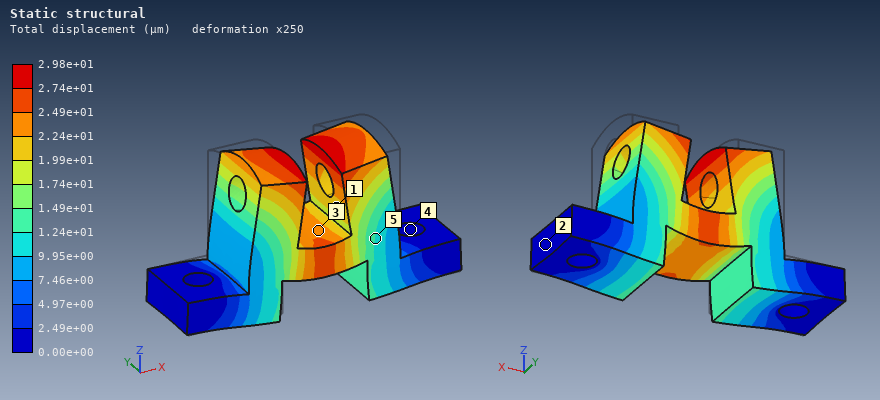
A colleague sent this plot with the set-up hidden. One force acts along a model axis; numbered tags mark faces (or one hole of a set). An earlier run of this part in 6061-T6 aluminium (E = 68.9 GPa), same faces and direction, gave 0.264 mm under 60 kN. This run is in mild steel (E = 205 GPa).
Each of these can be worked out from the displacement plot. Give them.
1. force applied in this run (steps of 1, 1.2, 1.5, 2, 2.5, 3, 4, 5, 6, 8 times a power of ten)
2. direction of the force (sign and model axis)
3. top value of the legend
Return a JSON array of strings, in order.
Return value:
["20 kN", "-Z", "2.98e+01 µm"]
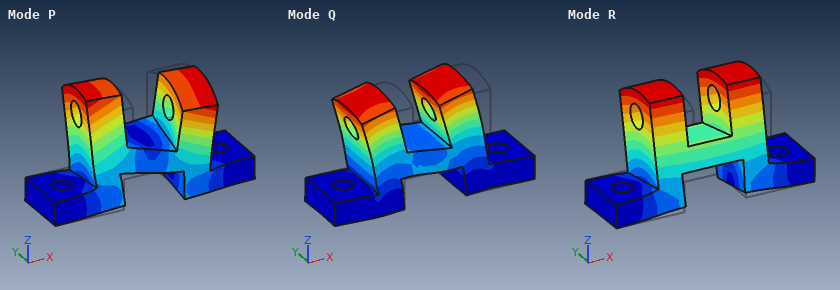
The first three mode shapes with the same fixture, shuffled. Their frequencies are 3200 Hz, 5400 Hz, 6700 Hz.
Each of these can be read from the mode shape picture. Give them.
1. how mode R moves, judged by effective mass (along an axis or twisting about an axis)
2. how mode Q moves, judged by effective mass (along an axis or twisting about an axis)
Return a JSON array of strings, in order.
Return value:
["along Y", "along X"]
